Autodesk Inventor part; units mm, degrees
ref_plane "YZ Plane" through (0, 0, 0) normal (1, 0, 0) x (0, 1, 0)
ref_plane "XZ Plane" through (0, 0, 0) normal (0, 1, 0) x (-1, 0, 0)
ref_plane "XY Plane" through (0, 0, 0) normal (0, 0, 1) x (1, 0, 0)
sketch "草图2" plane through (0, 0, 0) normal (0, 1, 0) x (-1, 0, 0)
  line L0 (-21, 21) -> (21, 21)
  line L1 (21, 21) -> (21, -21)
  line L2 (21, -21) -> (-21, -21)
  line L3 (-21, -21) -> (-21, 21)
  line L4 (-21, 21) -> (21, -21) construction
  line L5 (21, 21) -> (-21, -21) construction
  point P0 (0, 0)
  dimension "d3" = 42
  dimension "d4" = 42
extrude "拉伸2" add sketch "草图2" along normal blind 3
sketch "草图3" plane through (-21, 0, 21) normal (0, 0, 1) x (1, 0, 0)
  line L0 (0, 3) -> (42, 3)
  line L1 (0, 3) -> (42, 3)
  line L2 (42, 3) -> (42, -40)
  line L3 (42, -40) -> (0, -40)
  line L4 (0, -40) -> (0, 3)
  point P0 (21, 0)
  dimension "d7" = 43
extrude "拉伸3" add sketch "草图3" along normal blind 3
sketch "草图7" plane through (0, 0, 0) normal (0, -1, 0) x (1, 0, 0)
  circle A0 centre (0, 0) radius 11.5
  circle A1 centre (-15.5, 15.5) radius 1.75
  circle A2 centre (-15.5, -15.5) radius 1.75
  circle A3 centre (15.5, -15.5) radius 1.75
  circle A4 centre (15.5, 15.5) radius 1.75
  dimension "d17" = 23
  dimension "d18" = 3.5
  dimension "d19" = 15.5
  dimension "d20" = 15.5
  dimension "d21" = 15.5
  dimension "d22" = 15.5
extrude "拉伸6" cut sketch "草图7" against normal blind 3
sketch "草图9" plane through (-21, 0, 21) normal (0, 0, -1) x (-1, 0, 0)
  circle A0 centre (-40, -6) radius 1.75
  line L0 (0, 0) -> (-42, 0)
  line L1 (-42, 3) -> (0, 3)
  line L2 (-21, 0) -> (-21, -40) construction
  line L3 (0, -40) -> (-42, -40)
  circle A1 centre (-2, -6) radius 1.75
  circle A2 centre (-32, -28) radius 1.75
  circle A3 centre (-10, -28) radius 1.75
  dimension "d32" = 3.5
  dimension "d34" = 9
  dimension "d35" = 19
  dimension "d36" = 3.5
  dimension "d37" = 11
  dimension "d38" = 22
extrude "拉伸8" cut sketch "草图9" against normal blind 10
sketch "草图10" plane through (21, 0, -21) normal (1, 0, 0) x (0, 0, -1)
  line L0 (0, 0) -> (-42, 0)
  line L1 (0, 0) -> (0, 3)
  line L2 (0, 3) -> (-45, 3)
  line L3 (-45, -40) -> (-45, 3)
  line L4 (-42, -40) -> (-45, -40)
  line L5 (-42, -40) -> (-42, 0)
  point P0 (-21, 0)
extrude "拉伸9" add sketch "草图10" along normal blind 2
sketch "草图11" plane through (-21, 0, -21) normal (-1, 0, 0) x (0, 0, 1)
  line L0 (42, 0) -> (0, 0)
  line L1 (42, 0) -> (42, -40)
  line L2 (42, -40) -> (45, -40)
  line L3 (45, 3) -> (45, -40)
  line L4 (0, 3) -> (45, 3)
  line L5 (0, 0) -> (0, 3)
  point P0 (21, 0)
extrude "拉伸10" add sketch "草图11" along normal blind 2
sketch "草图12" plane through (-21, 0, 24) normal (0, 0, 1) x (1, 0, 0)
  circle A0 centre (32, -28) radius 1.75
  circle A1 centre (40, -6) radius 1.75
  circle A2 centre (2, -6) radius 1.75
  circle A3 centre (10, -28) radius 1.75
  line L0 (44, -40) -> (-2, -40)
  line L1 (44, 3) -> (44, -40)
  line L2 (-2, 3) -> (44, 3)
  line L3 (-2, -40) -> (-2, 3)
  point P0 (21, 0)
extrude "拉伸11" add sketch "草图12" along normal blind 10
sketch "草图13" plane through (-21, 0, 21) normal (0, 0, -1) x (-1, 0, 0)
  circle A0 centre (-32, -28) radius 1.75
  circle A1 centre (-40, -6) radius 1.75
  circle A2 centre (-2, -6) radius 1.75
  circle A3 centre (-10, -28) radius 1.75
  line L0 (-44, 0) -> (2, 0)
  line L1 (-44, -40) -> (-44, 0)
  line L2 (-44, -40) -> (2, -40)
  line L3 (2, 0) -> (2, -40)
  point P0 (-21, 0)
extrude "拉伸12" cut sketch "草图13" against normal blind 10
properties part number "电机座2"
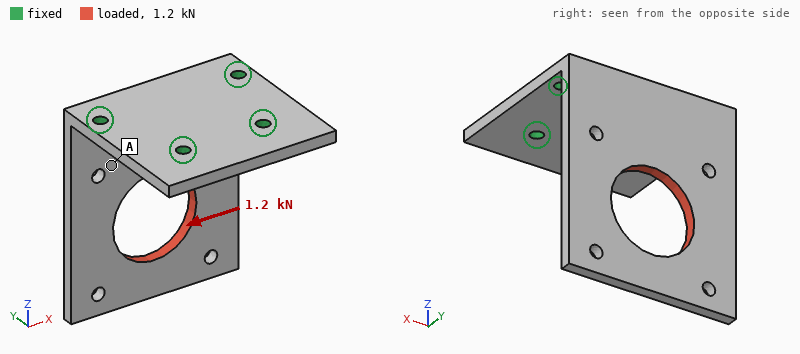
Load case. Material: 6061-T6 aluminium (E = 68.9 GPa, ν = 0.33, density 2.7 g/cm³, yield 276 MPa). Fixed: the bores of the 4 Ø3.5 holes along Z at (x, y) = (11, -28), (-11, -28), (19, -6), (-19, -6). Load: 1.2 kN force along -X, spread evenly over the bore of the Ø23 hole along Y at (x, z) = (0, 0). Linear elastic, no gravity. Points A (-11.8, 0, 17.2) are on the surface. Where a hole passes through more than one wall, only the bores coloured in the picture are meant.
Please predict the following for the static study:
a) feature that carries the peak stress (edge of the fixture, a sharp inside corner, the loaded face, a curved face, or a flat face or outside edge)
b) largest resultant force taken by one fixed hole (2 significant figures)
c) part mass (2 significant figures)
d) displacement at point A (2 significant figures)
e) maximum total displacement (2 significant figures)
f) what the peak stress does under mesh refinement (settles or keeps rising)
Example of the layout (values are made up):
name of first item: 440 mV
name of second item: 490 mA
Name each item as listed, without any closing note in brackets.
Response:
feature that carries the peak stress: edge of the fixture
largest resultant force taken by one fixed hole: 1.2 kN
part mass: 31 g
displacement at point A: 0.072 mm
maximum total displacement: 0.23 mm
what the peak stress does under mesh refinement: keeps rising
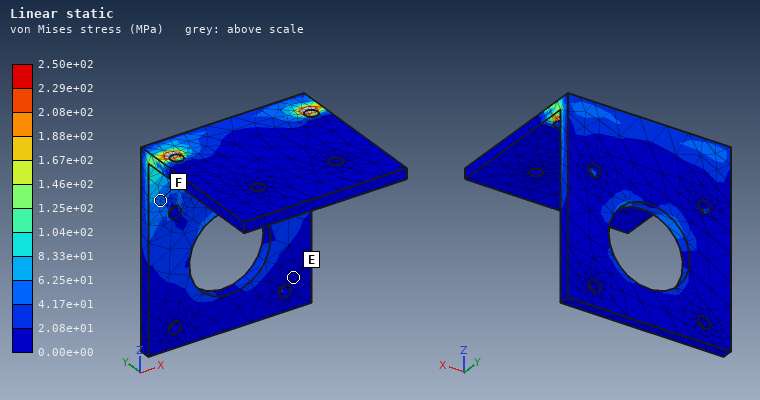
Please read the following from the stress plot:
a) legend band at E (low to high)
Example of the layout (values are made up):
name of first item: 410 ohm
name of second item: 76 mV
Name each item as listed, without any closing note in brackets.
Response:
legend band at E: 0.00e+00 to 2.08e+01 MPa
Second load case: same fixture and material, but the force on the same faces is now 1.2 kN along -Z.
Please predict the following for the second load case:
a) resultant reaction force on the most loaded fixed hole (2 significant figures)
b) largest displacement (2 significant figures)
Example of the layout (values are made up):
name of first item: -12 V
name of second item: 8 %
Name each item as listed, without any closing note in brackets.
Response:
resultant reaction force on the most loaded fixed hole: 650 N
largest displacement: 0.28 mm
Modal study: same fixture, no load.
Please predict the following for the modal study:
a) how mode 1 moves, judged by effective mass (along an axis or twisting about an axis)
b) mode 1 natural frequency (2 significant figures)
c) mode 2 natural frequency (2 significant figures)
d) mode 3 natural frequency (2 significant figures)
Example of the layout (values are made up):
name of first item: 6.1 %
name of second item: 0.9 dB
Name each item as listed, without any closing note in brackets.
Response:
how mode 1 moves, judged by effective mass: along Y
mode 1 natural frequency: 750 Hz
mode 2 natural frequency: 2000 Hz
mode 3 natural frequency: 4000 Hz
